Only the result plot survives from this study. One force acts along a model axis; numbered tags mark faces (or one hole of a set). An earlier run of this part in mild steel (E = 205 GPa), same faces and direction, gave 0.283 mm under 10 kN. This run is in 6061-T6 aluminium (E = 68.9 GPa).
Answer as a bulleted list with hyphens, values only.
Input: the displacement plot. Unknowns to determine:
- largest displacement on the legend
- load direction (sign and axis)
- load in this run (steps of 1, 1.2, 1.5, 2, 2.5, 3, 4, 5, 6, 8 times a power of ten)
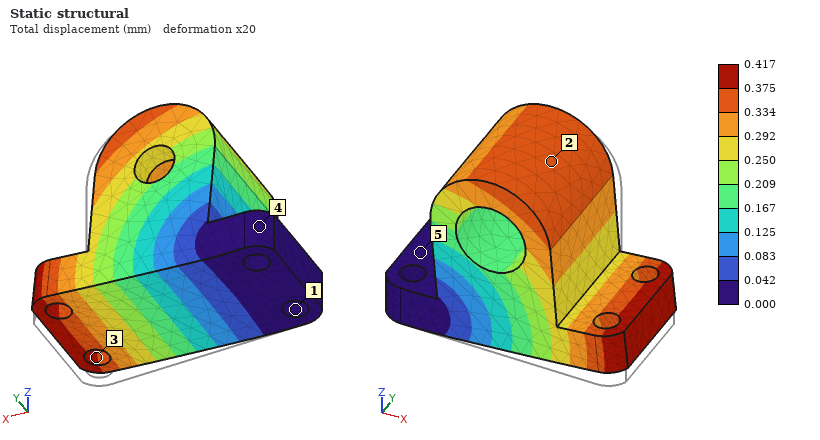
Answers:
- 0.417 mm
- +Z
- 5 kN
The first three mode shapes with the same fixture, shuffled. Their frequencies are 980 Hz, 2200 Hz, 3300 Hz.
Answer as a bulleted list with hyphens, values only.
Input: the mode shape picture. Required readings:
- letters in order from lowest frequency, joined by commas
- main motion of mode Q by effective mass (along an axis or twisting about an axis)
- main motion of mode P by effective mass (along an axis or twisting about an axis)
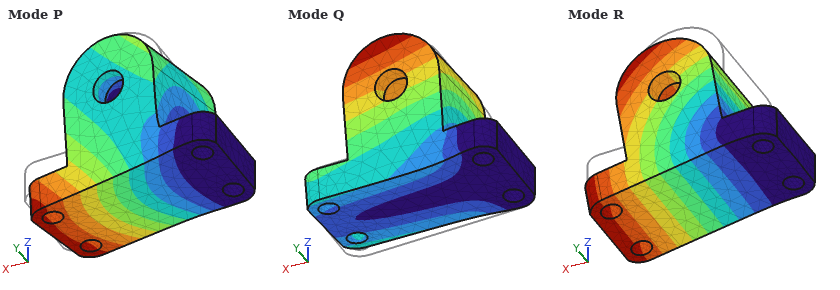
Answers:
- R, Q, P
- along Y
- along Y
